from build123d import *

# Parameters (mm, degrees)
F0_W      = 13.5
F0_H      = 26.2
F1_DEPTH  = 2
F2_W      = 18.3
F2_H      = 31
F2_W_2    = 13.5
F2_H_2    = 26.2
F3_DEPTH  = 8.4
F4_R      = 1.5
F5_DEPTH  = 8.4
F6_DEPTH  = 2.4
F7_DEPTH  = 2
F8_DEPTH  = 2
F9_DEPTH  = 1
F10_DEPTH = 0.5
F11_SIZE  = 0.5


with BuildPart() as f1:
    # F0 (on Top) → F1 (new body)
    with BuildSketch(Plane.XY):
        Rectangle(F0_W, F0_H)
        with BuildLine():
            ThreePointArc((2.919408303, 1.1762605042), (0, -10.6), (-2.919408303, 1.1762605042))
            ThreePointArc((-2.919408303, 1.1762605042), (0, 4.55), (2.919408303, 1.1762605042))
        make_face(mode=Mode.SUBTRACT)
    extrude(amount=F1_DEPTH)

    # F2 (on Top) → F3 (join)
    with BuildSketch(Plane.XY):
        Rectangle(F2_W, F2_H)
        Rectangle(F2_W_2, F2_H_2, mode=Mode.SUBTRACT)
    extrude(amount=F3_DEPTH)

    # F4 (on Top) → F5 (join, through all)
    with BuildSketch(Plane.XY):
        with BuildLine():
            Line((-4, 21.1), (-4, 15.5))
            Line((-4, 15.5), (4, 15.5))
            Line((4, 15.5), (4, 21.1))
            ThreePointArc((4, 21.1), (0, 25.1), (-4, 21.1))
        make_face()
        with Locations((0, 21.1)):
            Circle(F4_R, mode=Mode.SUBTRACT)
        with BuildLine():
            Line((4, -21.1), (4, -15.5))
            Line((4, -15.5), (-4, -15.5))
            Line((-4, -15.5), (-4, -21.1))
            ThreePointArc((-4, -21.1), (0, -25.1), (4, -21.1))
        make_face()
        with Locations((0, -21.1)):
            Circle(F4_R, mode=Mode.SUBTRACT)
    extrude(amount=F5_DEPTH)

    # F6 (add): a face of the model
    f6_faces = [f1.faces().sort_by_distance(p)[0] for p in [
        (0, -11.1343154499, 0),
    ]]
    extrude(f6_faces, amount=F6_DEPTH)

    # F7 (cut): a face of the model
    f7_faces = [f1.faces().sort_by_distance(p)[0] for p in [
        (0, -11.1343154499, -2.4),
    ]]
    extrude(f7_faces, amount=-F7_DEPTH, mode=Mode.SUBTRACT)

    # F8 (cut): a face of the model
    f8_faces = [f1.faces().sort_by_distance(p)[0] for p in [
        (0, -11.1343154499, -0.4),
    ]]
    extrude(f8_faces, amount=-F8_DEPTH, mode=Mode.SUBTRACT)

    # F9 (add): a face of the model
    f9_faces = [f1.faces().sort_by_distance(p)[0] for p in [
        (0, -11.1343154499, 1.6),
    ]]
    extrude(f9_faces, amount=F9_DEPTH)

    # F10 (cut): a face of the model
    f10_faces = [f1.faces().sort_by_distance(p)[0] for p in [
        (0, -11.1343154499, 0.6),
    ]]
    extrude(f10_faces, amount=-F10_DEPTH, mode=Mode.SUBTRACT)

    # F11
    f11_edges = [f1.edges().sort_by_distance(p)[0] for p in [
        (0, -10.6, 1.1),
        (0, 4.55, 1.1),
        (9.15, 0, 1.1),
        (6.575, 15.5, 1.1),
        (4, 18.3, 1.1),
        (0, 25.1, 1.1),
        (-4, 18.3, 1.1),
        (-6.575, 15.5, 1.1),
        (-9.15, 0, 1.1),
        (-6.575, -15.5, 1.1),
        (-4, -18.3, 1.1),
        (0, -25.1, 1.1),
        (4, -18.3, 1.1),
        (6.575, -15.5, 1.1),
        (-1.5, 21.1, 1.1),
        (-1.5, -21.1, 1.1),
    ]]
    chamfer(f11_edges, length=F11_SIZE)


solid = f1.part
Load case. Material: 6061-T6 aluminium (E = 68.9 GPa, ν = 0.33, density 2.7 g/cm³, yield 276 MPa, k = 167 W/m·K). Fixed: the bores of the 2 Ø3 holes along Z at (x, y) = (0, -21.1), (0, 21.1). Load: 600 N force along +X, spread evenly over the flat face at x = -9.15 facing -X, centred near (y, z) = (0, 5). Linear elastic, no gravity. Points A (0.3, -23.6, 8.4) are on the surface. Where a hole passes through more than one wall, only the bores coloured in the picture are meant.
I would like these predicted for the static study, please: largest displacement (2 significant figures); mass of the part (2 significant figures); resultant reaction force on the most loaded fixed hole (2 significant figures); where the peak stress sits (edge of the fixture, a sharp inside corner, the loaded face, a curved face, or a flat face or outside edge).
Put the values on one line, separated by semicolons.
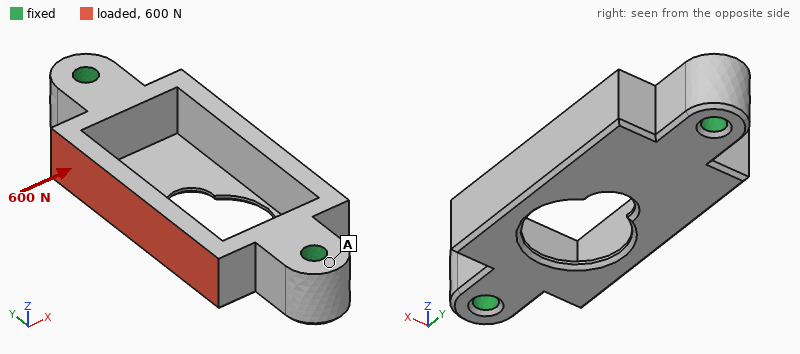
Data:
50 µm; 7.2 g; 370 N; a curved face
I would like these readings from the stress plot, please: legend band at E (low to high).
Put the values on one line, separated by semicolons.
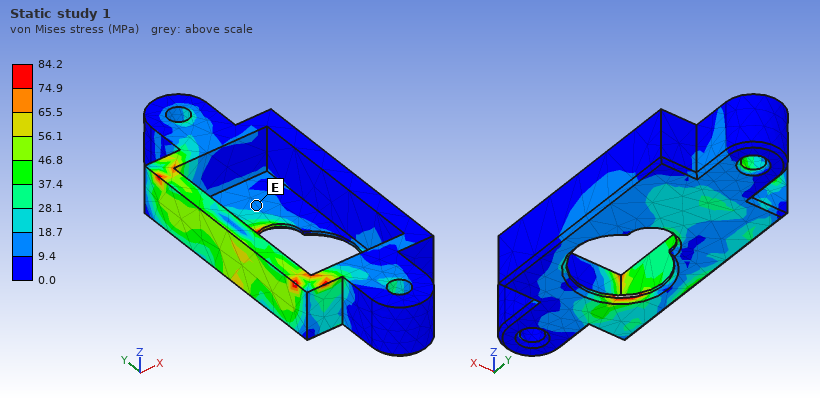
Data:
9.4 to 18.7 MPa
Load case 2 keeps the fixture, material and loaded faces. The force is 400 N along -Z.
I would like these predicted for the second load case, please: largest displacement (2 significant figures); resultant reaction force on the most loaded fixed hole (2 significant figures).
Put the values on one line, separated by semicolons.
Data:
36 µm; 200 N
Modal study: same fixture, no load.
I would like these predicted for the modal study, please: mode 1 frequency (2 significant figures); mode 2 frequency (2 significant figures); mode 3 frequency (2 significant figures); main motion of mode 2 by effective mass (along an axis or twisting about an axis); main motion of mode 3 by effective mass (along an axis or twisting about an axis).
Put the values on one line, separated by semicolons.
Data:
15 kHz; 17 kHz; 18 kHz; along Z; along X
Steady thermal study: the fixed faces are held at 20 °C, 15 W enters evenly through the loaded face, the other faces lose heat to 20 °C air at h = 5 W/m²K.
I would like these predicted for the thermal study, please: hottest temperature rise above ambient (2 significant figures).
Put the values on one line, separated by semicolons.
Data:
26 K
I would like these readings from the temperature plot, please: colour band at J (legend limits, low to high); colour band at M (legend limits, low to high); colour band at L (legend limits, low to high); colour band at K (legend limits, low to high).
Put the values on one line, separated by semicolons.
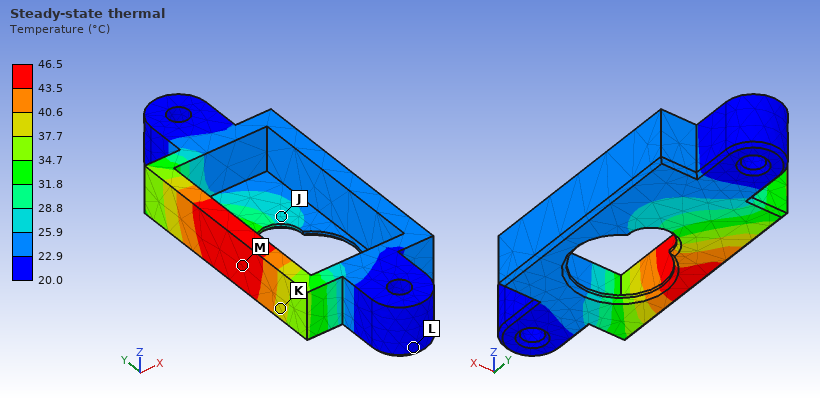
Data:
25.9 to 28.8 °C; 43.5 to 46.5 °C; 20.0 to 22.9 °C; 37.7 to 40.6 °C
